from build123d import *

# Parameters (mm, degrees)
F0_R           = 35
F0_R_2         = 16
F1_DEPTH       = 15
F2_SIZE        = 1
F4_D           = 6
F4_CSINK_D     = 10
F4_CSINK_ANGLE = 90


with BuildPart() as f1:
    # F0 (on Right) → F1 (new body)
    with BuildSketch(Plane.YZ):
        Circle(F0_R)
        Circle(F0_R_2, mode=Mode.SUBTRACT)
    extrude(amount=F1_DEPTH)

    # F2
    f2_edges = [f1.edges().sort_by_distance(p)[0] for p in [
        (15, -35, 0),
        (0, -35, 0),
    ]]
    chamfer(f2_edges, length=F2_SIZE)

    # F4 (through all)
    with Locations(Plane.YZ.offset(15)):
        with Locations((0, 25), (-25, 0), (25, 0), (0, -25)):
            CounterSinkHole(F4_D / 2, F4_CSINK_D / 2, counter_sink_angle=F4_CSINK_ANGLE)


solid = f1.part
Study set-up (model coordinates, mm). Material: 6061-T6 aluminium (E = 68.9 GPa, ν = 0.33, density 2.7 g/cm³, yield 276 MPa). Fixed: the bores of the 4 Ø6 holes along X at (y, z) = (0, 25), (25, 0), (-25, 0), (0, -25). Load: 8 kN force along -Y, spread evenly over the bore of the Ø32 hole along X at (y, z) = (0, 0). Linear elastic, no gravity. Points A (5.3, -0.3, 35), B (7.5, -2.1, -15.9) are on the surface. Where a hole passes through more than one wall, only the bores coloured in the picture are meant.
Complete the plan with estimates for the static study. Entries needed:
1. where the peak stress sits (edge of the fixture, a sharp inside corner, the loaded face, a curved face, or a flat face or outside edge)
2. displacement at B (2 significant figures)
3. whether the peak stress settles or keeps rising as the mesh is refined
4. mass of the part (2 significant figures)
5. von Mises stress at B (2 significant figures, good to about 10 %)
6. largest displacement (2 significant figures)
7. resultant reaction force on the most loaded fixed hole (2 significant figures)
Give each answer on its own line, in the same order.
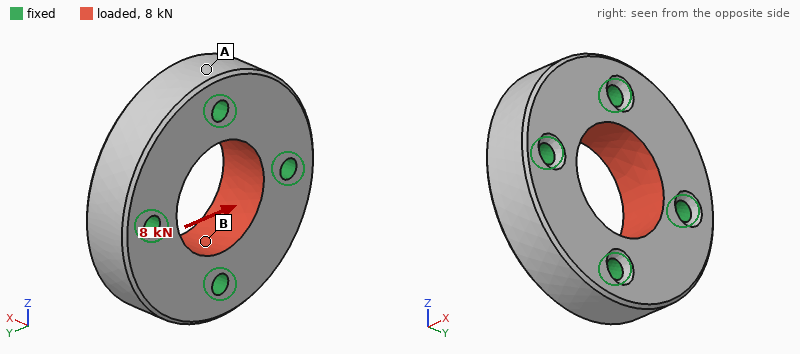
edge of the fixture
1.9 µm
keeps rising
120 g
9.0 MPa
2.2 µm
2.0 kN
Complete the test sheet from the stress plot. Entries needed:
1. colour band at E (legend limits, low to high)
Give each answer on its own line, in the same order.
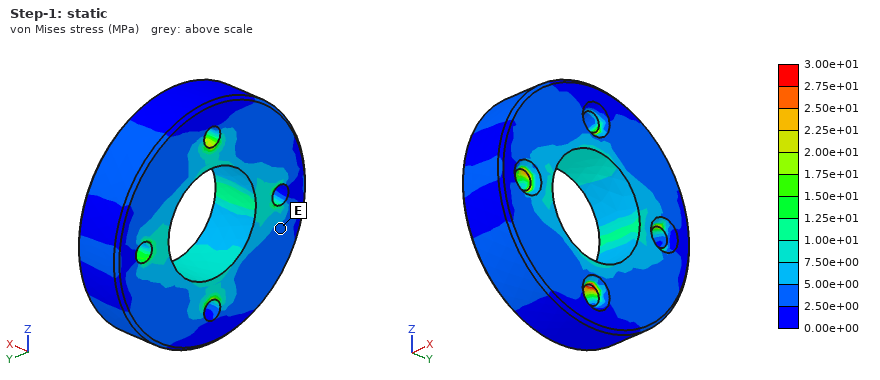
2.50e+00 to 5.00e+00 MPa
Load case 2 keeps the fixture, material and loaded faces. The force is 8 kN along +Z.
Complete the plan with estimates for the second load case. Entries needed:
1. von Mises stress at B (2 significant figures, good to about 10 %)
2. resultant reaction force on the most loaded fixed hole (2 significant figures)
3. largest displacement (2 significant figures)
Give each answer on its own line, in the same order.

11 MPa
2.0 kN
2.2 µm
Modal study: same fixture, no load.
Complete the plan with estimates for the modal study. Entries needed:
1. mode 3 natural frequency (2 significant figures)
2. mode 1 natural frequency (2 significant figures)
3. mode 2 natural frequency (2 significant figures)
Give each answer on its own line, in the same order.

24 kHz
22 kHz
24 kHz
